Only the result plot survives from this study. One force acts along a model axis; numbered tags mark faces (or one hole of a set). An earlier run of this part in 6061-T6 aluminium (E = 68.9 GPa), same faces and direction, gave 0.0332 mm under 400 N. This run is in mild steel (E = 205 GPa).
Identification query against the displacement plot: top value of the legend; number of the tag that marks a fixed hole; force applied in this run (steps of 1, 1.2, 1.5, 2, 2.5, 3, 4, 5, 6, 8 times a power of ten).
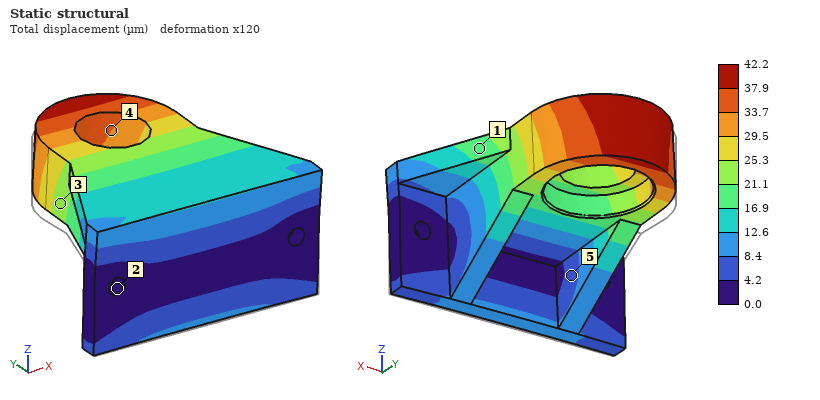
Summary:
42.2 µm
2
1.5 kN
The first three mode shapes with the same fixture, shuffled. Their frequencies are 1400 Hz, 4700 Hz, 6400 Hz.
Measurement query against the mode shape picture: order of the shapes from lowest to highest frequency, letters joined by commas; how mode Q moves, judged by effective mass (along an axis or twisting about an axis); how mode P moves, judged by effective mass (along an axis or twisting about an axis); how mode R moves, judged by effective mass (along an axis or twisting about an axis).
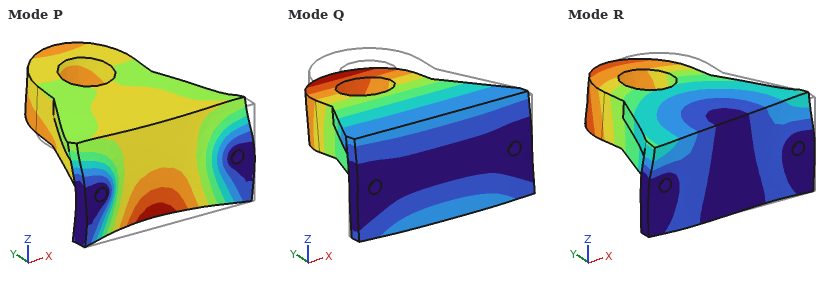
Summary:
Q, R, P
along Z
along Y
along X
